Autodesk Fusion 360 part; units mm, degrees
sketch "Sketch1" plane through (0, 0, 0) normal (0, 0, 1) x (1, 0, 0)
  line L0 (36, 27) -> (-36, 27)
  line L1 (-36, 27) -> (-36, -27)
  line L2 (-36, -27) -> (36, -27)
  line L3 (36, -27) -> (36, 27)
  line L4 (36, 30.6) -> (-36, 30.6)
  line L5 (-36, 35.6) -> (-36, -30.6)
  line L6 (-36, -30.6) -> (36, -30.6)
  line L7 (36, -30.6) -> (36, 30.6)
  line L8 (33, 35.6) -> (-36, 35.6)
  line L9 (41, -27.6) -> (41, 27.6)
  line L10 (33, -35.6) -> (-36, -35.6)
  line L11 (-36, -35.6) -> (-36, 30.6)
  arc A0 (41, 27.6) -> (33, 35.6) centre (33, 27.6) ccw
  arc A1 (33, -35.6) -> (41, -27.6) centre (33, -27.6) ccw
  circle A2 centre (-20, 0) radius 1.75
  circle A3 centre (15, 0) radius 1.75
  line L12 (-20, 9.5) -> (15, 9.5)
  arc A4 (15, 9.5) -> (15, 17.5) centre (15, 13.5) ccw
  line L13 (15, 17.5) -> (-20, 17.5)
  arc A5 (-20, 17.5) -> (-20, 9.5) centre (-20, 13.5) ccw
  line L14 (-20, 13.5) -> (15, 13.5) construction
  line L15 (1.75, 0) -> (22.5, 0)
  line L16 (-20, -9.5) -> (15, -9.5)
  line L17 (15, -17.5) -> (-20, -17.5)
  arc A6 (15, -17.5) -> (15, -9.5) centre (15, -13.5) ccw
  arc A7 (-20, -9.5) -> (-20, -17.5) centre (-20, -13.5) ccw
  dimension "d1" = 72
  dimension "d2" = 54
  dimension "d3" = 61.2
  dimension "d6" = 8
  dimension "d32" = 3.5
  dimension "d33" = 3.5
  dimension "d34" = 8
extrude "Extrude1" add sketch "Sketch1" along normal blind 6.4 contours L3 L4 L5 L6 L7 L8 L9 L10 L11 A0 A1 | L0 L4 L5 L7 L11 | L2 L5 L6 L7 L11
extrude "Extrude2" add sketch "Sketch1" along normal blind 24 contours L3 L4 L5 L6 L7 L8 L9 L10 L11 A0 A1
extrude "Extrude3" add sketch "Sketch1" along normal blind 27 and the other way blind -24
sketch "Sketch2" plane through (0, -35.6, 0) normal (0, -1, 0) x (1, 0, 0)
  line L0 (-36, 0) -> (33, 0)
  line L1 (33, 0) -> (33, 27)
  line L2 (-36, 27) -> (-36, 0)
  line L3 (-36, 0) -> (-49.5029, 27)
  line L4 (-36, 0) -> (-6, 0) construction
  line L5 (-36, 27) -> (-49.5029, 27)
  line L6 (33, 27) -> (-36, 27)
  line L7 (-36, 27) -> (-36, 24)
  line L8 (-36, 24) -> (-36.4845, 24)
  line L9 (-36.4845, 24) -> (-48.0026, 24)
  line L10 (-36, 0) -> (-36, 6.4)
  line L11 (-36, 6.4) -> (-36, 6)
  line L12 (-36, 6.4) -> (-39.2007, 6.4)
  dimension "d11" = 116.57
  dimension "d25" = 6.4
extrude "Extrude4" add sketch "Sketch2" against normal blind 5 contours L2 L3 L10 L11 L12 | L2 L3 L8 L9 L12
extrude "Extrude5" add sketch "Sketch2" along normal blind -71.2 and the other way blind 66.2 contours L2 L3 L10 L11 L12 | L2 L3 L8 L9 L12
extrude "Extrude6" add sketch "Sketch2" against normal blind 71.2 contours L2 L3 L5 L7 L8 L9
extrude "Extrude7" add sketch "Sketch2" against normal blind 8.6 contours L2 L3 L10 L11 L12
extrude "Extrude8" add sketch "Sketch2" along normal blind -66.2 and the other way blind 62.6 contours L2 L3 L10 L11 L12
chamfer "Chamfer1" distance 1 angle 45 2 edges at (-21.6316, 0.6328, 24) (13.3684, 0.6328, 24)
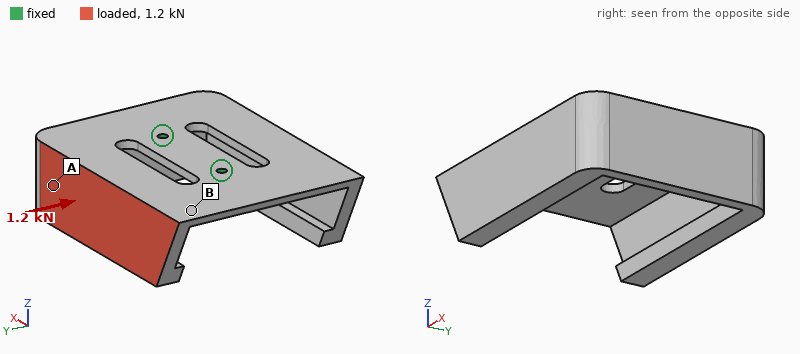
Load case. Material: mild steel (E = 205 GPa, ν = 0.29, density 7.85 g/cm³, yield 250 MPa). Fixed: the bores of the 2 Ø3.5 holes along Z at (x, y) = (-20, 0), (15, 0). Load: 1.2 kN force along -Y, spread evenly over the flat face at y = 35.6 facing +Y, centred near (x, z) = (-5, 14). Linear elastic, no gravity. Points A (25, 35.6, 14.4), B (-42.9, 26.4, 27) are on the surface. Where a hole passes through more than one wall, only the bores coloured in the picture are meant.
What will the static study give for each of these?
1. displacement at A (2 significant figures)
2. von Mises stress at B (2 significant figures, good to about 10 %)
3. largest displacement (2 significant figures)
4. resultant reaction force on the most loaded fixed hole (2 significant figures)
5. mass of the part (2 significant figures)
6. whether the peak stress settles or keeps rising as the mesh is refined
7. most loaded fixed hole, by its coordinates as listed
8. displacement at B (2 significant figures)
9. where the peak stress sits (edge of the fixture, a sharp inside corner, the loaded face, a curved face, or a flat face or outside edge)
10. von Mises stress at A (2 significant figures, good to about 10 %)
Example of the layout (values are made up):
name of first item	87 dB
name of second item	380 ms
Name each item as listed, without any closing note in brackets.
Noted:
displacement at A	0.30 mm
von Mises stress at B	68 MPa
largest displacement	0.38 mm
resultant reaction force on the most loaded fixed hole	700 N
mass of the part	370 g
whether the peak stress settles or keeps rising as the mesh is refined	keeps rising
most loaded fixed hole, by its coordinates as listed	(-20, 0)
displacement at B	0.17 mm
where the peak stress sits	edge of the fixture
von Mises stress at A	36 MPa
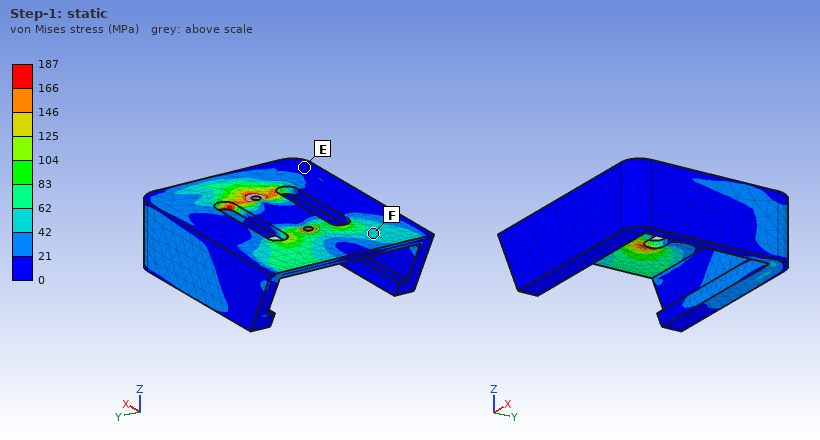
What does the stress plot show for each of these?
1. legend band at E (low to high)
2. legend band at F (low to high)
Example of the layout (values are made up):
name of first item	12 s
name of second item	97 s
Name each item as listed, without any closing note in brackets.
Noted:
legend band at E	0 to 21 MPa
legend band at F	42 to 62 MPa
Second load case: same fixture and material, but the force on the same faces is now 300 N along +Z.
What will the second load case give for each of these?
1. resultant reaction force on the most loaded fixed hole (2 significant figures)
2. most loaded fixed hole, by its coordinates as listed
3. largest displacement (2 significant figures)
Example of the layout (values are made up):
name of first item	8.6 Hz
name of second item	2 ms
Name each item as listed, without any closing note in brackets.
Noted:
resultant reaction force on the most loaded fixed hole	180 N
most loaded fixed hole, by its coordinates as listed	(-20, 0)
largest displacement	0.25 mm
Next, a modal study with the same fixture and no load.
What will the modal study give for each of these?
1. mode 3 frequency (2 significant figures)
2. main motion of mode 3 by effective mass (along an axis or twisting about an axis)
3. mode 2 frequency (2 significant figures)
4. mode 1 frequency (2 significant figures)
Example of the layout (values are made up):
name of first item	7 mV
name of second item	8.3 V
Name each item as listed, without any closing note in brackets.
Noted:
mode 3 frequency	1200 Hz
main motion of mode 3 by effective mass	along Z
mode 2 frequency	950 Hz
mode 1 frequency	410 Hz
